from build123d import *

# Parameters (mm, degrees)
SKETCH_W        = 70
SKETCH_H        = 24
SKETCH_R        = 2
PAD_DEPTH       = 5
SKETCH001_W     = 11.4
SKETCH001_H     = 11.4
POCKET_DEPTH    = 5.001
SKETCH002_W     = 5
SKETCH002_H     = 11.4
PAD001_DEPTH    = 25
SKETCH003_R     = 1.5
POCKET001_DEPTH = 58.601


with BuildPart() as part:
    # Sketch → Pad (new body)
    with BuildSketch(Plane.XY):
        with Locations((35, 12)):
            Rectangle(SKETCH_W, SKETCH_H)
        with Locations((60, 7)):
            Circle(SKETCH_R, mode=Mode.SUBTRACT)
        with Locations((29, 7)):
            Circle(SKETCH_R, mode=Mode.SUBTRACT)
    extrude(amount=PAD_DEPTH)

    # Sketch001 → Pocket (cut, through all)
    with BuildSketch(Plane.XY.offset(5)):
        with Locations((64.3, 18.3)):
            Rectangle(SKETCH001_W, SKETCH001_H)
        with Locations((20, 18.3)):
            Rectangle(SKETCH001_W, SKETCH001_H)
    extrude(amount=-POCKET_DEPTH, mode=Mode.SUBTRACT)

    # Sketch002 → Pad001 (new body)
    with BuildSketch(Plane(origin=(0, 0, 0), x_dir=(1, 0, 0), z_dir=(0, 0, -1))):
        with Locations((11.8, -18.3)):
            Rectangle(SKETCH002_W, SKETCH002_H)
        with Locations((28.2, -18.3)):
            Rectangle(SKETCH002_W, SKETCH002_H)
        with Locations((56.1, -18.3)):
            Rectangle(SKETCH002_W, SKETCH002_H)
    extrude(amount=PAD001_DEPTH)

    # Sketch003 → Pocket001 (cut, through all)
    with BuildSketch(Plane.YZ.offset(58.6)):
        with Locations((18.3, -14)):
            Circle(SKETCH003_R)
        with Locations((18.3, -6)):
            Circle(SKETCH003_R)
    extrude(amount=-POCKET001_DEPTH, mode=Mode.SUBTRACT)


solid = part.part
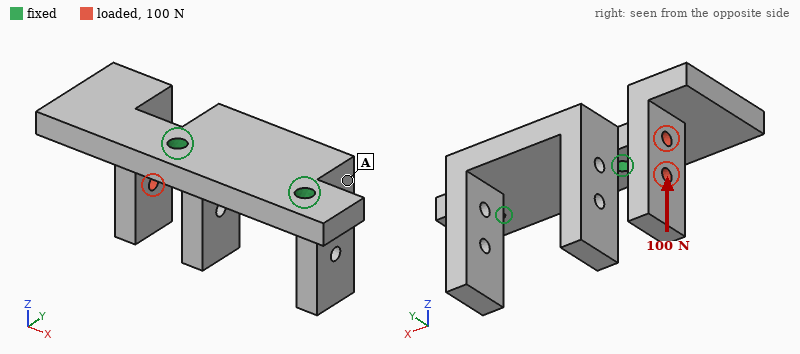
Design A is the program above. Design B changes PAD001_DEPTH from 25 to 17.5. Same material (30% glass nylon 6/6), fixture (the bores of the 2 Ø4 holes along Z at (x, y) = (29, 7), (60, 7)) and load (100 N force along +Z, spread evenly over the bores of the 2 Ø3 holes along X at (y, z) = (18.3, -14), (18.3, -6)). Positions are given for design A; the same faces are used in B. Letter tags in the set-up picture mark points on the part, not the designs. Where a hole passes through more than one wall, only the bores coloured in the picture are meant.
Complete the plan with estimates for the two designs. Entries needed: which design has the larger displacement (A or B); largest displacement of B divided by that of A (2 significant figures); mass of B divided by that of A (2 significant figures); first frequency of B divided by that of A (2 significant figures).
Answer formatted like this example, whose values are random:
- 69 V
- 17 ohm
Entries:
- A
- 0.84
- 0.88
- 1.2
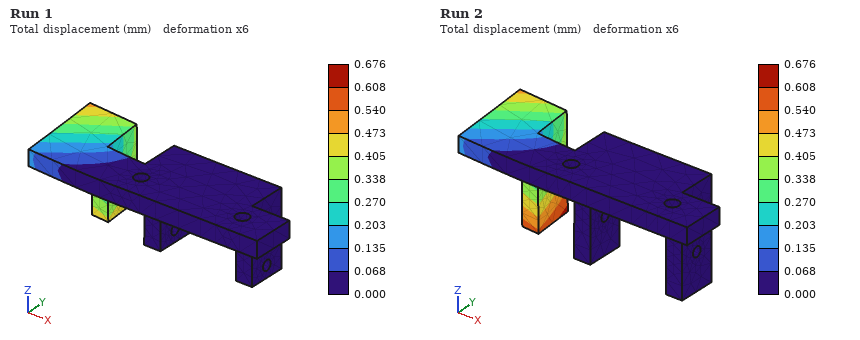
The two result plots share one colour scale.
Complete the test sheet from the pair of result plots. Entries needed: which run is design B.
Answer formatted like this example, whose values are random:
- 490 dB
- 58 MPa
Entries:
- Run 1
